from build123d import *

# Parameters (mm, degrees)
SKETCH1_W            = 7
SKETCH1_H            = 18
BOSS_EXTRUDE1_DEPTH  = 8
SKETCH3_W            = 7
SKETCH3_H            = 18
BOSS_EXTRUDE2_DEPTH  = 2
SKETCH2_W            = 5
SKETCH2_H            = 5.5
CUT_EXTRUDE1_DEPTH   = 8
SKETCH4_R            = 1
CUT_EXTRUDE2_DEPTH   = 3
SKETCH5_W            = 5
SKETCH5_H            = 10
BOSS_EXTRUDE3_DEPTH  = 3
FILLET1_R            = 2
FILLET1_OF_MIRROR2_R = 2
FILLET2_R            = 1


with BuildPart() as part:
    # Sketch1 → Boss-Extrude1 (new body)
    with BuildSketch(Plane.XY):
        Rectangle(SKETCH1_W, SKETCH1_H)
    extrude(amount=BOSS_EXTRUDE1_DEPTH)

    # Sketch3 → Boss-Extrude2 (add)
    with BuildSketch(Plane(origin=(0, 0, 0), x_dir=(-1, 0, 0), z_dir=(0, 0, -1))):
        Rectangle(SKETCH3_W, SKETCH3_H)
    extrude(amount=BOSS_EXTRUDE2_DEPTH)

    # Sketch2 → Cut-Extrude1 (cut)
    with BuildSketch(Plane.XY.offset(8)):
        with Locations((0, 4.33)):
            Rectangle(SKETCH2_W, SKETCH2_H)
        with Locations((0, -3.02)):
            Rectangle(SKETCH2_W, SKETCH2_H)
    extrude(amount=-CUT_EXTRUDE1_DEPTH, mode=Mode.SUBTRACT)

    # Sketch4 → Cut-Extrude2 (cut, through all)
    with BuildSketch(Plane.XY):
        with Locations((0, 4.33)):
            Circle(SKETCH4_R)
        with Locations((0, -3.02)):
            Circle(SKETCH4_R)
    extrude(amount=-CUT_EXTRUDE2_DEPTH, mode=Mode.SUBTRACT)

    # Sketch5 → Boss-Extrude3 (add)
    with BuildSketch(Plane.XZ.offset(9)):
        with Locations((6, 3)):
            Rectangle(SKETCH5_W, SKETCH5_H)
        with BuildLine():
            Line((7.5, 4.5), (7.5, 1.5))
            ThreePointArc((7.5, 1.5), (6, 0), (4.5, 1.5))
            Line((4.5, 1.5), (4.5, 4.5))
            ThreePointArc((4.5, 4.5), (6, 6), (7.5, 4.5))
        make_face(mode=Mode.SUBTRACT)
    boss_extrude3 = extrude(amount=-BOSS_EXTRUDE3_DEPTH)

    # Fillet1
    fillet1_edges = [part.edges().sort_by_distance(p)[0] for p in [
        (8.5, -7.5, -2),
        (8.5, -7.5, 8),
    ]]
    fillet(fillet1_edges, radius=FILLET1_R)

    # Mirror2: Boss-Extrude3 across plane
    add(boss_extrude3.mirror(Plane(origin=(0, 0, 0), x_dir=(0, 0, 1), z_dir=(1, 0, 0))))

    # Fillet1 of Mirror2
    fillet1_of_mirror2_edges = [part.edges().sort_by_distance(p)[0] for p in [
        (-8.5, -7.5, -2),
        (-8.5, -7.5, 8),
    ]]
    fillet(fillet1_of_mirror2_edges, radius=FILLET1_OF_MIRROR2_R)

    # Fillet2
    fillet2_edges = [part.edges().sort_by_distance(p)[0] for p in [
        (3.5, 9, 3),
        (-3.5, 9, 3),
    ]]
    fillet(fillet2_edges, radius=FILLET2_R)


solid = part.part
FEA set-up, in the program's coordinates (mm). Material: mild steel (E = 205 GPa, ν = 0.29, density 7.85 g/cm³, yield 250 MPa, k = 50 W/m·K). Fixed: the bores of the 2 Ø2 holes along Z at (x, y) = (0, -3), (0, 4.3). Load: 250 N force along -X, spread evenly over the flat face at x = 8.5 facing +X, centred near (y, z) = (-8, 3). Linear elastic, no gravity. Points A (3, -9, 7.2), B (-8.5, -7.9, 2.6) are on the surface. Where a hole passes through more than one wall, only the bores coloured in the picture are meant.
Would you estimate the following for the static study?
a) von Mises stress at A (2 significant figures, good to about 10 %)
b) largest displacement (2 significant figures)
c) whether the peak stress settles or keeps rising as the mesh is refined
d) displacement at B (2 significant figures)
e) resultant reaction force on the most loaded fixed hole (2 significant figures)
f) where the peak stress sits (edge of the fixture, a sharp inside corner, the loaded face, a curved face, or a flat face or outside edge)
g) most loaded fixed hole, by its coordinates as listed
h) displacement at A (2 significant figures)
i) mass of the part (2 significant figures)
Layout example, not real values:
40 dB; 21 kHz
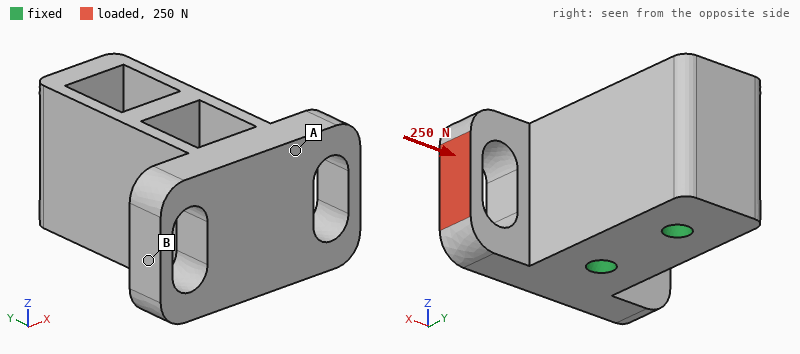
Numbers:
28 MPa; 12 µm; keeps rising; 7.7 µm; 330 N; edge of the fixture; (0, -3); 8.5 µm; 7.8 g
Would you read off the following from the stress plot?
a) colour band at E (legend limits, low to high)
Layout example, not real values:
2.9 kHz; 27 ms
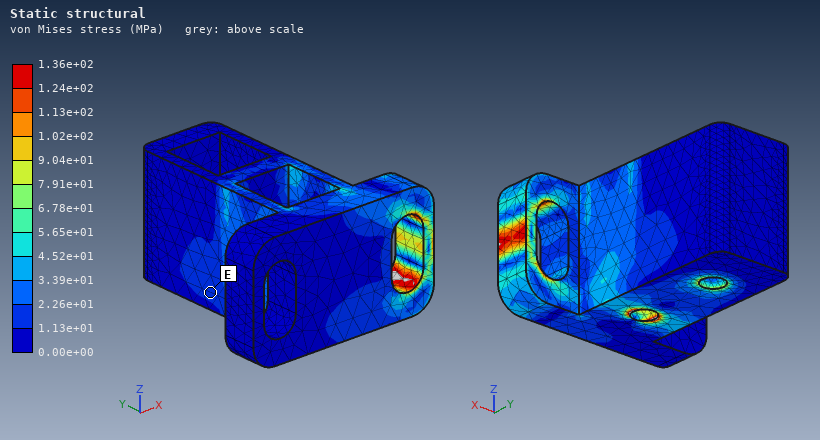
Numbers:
1.13e+01 to 2.26e+01 MPa
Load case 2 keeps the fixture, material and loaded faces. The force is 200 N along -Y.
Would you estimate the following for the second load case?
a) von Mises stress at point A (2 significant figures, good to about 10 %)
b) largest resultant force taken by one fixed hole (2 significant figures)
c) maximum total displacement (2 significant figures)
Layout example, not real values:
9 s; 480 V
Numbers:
87 MPa; 210 N; 17 µm
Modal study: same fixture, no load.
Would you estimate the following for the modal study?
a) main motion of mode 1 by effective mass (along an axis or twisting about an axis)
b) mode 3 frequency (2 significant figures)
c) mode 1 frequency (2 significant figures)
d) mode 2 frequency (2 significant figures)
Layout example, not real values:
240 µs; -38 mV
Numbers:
along X; 25 kHz; 13 kHz; 22 kHz
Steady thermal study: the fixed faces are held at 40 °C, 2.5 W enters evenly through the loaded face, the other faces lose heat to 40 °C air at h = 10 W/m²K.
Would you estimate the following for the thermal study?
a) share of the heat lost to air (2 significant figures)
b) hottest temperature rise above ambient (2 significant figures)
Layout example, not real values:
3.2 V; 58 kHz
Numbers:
3.4 %; 42 K
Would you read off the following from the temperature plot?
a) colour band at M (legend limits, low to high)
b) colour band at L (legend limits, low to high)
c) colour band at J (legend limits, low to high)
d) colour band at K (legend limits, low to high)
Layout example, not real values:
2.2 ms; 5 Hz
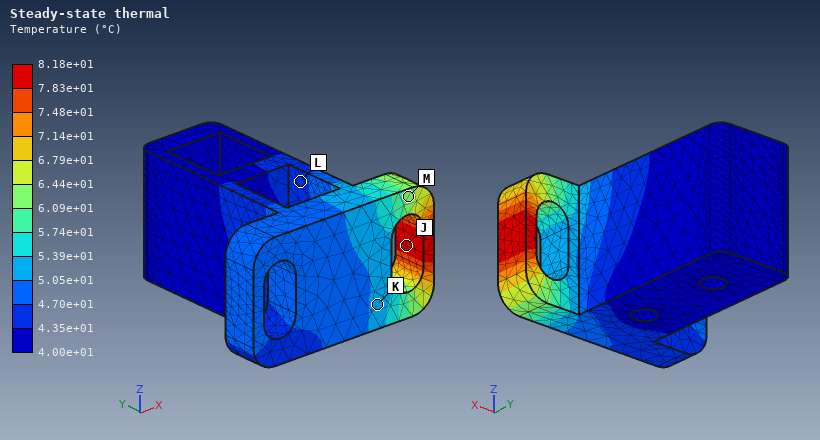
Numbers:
6.09e+01 to 6.44e+01 °C; 4.35e+01 to 4.70e+01 °C; 7.83e+01 to 8.18e+01 °C; 5.05e+01 to 5.39e+01 °C
